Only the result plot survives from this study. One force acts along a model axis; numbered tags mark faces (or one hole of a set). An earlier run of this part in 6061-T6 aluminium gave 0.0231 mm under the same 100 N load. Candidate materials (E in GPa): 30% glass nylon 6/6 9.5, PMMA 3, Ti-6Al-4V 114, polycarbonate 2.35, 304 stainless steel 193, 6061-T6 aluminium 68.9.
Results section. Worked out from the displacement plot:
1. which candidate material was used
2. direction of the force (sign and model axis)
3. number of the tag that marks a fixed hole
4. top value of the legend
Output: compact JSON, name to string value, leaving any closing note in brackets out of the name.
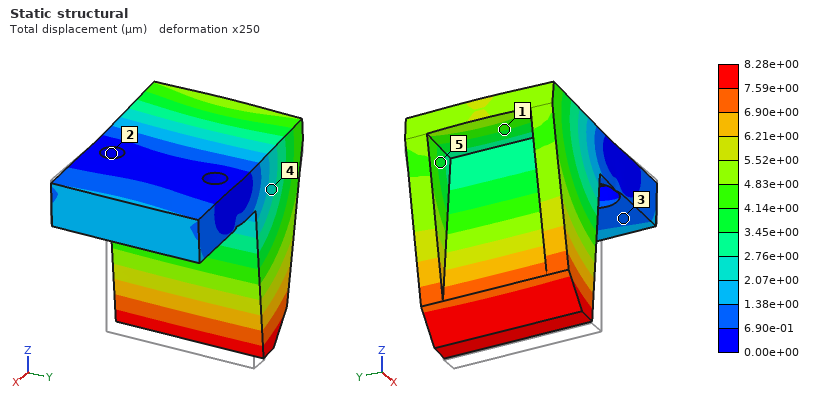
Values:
{"which candidate material was used": "304 stainless steel", "direction of the force": "+Z", "number of the tag that marks a fixed hole": "2", "top value of the legend": "8.28e+00 µm"}
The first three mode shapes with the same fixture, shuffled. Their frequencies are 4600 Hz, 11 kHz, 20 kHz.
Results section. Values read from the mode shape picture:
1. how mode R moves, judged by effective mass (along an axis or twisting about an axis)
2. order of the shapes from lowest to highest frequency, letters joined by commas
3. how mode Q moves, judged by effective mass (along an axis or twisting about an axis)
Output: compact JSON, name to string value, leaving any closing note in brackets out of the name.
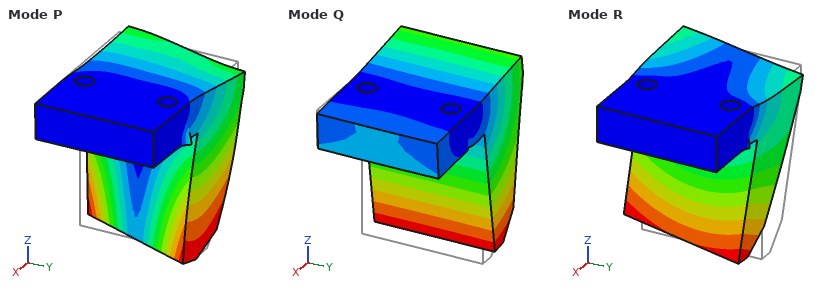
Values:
{"how mode R moves, judged by effective mass": "along Y", "order of the shapes from lowest to highest frequency, letters joined by commas": "Q, R, P", "how mode Q moves, judged by effective mass": "along X"}
